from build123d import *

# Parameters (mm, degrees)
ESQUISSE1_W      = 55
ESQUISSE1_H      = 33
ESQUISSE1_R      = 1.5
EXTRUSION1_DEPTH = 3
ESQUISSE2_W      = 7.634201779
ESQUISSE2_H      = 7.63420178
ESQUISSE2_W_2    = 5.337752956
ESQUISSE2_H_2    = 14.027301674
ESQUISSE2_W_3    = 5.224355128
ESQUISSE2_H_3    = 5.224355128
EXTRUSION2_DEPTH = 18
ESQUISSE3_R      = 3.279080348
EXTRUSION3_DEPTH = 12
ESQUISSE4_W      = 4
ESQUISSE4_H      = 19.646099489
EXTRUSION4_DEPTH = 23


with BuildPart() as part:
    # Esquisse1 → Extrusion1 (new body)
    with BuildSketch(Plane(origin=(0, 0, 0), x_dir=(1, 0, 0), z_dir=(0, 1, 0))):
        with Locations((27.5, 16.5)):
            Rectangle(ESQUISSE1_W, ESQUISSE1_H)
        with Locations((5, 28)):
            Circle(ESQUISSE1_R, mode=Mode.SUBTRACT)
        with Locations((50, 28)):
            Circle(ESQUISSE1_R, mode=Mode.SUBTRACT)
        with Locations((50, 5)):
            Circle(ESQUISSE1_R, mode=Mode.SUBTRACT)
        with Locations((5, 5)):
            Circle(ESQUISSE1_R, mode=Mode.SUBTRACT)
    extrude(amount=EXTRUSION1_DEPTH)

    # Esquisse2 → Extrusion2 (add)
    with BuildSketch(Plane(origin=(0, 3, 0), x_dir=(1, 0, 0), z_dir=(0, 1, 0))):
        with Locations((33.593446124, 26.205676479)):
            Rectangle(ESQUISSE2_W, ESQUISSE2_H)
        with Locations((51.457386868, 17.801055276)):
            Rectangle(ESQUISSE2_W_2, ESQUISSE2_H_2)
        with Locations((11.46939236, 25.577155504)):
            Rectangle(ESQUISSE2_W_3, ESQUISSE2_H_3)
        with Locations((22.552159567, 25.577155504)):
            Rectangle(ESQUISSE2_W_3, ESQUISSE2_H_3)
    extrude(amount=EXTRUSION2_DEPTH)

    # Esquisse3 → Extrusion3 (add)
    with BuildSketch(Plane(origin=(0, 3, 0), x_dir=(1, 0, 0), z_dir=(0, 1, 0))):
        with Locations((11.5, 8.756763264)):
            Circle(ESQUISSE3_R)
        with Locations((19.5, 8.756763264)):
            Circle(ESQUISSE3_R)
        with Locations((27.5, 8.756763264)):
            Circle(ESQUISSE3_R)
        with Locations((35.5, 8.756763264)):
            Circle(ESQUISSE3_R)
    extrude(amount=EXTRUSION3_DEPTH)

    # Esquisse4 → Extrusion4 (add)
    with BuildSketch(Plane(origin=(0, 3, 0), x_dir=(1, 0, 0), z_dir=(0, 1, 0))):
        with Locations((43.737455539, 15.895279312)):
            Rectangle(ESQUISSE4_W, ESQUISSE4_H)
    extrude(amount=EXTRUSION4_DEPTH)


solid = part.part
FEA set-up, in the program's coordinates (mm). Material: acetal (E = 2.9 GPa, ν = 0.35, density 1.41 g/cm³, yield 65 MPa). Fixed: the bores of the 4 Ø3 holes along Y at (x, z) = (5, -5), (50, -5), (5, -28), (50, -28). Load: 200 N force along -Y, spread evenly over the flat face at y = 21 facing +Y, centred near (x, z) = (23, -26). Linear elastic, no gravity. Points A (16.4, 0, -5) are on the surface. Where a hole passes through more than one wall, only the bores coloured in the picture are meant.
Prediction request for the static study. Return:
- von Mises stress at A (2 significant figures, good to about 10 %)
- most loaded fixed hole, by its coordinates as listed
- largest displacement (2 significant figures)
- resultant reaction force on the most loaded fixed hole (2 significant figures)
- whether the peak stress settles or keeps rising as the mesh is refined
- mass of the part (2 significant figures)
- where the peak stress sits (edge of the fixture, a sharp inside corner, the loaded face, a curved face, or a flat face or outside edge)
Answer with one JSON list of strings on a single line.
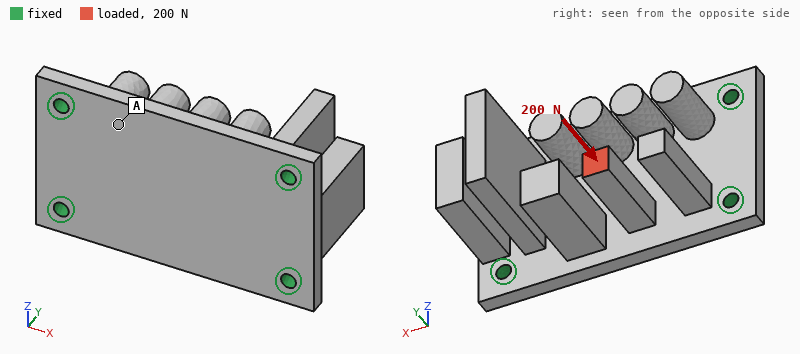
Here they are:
["3.4 MPa", "(5, -28)", "0.79 mm", "110 N", "keeps rising", "17 g", "edge of the fixture"]
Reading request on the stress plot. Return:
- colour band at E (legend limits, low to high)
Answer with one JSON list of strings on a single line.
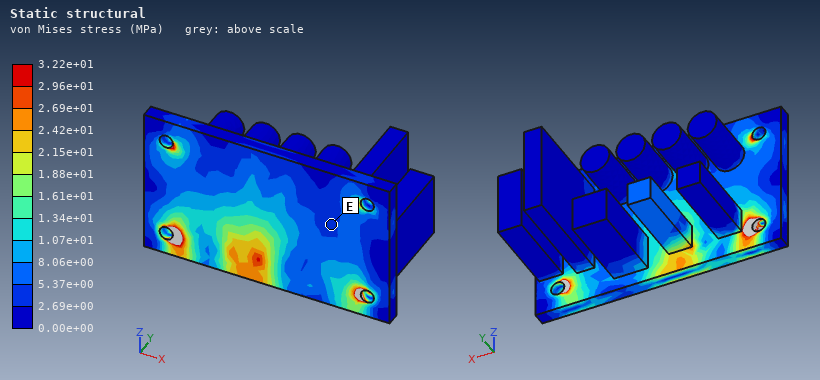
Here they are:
["2.69e+00 to 5.37e+00 MPa"]
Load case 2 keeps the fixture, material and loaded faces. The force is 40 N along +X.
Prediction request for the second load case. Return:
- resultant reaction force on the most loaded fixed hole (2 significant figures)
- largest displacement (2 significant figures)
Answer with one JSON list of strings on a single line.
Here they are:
["27 N", "0.81 mm"]
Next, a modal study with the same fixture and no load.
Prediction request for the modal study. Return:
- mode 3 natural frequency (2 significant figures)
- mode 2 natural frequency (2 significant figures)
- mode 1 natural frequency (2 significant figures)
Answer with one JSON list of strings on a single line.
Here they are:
["1700 Hz", "1500 Hz", "1100 Hz"]
